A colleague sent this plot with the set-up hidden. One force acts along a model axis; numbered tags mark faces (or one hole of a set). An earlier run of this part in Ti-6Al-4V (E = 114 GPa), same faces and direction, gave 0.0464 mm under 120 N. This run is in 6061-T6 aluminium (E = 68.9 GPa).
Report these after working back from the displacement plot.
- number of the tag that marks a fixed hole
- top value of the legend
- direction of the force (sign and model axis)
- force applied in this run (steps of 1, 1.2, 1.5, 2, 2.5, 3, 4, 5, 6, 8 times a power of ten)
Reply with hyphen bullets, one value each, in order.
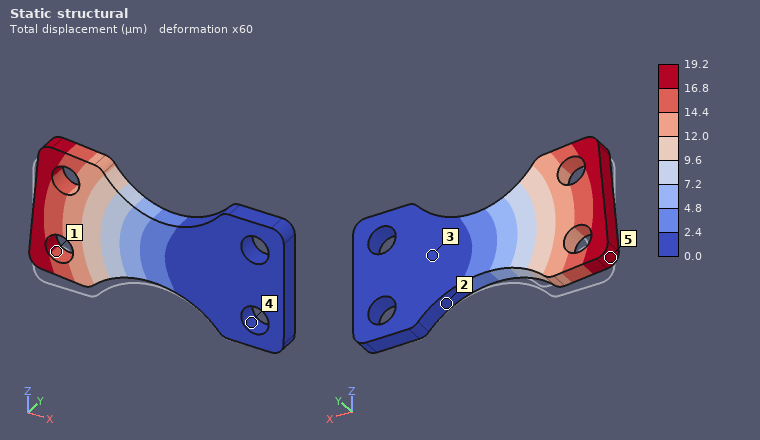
- 4
- 19.2 µm
- +Z
- 30 N
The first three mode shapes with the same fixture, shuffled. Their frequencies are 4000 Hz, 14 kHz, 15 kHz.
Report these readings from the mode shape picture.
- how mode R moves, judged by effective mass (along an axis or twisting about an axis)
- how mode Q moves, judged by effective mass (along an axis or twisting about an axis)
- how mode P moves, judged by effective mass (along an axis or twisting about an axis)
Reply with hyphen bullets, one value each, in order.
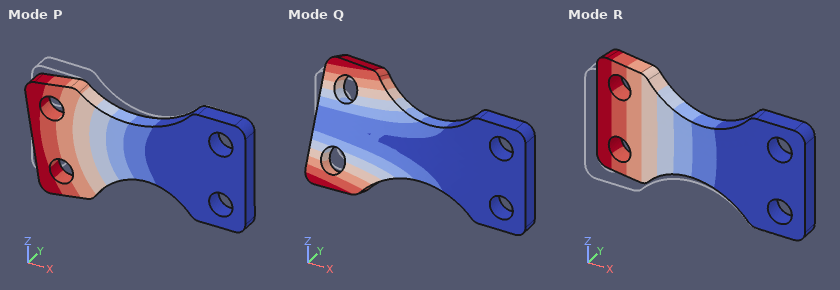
- along Y
- twisting about X
- along Z
